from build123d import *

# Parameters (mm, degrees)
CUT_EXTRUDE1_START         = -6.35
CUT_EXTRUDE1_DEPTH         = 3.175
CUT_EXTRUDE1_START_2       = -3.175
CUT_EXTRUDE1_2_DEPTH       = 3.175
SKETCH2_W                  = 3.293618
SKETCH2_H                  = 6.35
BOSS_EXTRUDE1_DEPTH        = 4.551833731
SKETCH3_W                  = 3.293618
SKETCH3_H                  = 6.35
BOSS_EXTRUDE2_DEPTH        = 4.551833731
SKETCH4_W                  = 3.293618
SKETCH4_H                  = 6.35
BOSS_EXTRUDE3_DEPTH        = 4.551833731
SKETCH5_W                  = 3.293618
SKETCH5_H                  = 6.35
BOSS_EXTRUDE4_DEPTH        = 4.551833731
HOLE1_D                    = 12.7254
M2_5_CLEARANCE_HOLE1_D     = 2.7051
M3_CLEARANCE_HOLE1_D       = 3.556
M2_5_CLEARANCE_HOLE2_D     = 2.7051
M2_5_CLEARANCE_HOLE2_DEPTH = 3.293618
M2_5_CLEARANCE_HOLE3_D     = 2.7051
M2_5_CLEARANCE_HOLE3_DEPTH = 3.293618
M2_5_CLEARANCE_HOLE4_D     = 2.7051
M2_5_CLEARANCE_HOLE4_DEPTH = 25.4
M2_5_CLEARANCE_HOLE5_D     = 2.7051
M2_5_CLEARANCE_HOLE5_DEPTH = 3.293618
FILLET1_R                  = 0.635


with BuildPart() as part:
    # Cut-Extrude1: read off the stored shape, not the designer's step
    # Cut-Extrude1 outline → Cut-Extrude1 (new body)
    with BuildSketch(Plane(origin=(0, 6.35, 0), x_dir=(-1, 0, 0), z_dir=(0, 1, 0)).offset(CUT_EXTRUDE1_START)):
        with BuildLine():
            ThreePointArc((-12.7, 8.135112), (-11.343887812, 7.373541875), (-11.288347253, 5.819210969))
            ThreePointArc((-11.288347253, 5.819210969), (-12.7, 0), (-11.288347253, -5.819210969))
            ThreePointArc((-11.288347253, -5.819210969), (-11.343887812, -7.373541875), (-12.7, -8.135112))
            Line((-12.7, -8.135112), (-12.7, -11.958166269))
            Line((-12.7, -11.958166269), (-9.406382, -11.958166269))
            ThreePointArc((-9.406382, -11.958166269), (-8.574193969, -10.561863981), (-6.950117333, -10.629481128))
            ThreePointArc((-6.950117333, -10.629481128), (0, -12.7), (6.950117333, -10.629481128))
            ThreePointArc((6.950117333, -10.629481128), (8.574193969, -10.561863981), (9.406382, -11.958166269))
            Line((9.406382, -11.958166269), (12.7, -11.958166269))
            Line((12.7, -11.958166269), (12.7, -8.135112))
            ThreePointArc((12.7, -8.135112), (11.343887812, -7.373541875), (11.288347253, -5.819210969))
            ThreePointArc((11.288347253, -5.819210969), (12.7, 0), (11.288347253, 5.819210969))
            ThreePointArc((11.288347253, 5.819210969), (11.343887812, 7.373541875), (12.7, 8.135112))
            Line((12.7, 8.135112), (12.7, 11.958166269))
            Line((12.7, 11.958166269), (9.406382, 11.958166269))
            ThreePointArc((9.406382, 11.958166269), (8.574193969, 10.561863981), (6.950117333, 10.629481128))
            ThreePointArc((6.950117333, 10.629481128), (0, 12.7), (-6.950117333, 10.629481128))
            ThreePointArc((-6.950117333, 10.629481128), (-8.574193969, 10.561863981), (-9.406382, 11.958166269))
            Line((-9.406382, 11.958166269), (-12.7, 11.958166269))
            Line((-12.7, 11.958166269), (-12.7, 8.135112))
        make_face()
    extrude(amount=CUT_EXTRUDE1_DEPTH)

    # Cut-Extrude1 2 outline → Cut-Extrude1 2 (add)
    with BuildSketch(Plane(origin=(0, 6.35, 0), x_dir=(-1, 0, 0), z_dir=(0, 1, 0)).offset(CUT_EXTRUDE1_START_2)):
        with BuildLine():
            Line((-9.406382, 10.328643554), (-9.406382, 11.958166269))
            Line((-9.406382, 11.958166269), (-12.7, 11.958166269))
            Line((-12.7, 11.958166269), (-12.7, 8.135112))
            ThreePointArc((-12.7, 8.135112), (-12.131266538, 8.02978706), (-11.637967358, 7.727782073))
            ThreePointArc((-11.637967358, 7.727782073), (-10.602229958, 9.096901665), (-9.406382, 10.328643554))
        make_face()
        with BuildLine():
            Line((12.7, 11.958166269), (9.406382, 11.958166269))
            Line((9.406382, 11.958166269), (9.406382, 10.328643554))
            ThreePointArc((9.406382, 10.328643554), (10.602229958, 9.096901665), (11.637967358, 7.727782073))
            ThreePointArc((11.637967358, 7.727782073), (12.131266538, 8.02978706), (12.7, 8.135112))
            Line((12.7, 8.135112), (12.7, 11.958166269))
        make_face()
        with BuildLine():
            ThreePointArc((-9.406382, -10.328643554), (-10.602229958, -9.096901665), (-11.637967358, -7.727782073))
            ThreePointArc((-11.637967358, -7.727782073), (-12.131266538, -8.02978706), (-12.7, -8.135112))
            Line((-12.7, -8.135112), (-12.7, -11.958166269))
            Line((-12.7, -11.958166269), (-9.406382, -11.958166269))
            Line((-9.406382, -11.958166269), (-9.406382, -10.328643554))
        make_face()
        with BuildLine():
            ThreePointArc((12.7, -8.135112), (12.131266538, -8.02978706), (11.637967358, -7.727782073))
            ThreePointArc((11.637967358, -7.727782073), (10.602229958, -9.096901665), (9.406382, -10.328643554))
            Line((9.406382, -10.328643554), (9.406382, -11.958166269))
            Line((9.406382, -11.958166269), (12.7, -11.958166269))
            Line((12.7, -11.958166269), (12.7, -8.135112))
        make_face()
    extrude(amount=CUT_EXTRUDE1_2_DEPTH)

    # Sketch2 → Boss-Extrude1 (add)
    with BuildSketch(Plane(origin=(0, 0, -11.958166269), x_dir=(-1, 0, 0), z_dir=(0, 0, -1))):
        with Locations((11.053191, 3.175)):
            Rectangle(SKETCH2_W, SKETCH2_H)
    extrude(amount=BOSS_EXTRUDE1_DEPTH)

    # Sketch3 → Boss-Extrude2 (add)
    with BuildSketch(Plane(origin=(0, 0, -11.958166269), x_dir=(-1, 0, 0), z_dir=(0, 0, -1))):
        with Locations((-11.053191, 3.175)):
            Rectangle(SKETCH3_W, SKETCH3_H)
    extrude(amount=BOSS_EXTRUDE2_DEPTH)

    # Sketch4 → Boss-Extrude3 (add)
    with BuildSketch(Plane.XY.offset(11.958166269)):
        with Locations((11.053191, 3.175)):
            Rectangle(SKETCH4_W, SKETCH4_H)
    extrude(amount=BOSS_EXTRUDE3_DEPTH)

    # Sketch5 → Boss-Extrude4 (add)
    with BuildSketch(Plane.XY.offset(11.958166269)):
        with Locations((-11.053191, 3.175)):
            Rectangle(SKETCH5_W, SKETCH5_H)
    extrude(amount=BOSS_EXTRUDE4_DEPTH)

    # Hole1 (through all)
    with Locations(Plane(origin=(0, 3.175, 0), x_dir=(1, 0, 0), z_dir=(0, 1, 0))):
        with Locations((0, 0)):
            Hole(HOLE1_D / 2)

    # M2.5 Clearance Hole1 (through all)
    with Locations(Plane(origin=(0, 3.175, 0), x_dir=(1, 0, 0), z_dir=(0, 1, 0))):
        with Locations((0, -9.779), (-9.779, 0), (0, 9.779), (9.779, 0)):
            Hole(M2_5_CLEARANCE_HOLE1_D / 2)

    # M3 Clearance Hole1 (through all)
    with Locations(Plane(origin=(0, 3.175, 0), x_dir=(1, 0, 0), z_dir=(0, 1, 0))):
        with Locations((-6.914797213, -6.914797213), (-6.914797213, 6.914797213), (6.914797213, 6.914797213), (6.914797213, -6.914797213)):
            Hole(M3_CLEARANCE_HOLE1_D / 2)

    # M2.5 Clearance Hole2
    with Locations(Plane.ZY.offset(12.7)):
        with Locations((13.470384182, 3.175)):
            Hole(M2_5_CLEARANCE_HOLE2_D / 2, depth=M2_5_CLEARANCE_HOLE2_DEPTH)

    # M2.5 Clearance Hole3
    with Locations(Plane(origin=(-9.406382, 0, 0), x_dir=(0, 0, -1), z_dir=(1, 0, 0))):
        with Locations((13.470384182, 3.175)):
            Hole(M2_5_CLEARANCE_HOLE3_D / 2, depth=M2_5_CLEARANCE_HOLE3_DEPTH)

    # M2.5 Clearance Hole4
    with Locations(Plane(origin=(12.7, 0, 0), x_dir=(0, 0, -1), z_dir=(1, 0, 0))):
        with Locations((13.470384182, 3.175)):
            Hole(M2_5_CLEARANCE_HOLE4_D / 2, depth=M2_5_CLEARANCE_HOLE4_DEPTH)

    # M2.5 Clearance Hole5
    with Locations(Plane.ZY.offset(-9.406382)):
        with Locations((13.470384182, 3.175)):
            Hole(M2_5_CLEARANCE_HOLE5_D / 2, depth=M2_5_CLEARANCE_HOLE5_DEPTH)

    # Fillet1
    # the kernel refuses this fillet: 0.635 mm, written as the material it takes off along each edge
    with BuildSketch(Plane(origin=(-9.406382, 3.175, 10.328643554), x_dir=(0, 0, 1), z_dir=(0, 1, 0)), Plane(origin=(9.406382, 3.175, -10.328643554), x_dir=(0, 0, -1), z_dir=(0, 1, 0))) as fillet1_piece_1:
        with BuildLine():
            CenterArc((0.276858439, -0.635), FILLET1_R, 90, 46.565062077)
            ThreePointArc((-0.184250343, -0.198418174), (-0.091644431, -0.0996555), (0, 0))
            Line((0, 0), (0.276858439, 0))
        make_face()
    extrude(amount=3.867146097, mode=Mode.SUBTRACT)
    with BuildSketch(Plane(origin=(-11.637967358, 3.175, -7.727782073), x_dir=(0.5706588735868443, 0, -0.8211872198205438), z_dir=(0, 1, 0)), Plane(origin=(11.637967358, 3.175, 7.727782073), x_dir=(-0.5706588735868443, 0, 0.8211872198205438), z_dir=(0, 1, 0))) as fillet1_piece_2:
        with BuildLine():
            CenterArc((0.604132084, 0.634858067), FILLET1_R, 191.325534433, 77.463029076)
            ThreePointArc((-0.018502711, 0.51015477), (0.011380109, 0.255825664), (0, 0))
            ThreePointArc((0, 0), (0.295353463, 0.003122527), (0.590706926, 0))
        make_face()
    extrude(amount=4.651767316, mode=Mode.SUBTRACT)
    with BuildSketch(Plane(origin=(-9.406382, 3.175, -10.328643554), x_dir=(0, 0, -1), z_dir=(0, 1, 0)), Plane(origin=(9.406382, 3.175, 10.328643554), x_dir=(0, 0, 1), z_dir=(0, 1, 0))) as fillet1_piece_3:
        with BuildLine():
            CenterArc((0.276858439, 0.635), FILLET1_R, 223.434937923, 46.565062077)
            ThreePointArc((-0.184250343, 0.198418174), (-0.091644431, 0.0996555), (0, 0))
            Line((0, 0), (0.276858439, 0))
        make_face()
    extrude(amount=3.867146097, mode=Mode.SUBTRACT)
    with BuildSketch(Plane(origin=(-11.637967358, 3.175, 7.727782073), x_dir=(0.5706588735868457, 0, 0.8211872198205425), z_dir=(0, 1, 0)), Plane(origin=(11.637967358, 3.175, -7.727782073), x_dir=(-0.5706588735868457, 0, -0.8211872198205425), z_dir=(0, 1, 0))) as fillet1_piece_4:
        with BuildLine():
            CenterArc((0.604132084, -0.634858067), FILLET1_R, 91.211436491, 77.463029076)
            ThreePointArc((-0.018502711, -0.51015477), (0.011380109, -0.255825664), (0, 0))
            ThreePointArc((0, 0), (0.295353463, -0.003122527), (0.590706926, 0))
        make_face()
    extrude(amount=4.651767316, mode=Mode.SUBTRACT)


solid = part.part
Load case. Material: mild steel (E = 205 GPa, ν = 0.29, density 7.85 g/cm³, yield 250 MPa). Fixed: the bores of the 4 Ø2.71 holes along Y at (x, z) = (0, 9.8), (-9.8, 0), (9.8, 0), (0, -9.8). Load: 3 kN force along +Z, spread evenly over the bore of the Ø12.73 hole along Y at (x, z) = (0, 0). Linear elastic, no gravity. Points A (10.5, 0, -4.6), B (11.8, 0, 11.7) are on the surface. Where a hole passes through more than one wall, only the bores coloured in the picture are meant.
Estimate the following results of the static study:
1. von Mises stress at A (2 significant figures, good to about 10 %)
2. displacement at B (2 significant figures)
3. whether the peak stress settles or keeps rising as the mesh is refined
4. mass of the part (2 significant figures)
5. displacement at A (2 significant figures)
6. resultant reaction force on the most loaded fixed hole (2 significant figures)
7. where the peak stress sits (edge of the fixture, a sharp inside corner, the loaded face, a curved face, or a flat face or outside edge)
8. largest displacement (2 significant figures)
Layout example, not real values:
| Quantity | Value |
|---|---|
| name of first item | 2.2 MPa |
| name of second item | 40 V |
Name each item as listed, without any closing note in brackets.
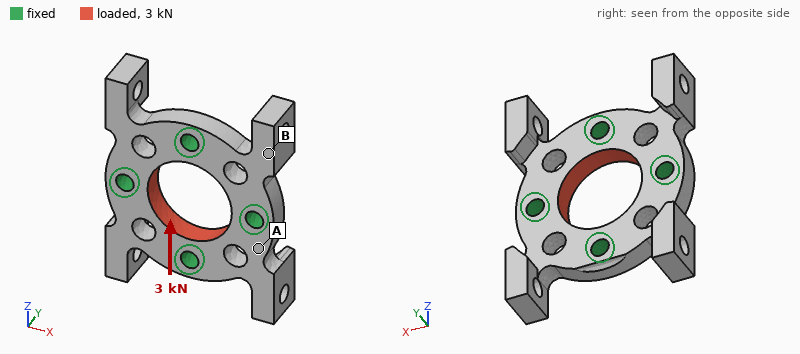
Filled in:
| Quantity | Value |
|---|---|
| von Mises stress at A | 19 MPa |
| displacement at B | 0.56 µm |
| whether the peak stress settles or keeps rising as the mesh is refined | keeps rising |
| mass of the part | 13 g |
| displacement at A | 0.61 µm |
| resultant reaction force on the most loaded fixed hole | 770 N |
| where the peak stress sits | edge of the fixture |
| largest displacement | 1.7 µm |
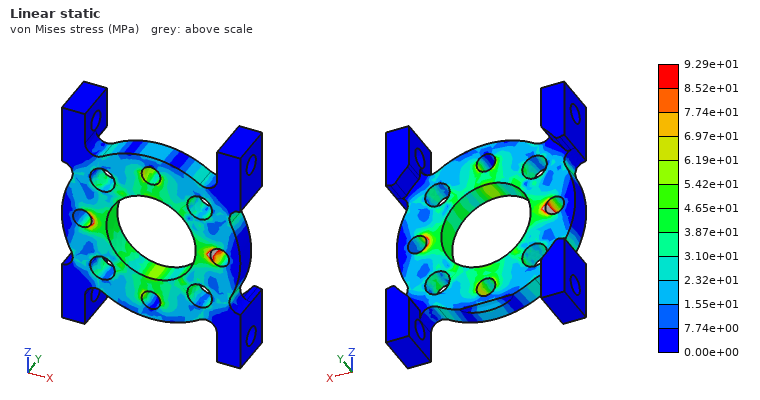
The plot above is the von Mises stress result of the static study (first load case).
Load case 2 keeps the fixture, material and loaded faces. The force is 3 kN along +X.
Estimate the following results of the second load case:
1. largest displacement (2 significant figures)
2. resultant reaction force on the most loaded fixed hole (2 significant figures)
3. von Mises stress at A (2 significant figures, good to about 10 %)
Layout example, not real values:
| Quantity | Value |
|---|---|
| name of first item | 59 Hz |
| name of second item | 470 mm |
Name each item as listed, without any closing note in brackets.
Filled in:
| Quantity | Value |
|---|---|
| largest displacement | 1.7 µm |
| resultant reaction force on the most loaded fixed hole | 760 N |
| von Mises stress at A | 17 MPa |
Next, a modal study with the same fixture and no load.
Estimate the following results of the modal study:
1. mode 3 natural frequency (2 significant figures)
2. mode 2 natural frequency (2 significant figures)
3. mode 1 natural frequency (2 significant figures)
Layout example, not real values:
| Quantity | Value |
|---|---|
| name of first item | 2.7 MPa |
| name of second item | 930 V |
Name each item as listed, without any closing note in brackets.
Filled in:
| Quantity | Value |
|---|---|
| mode 3 natural frequency | 12 kHz |
| mode 2 natural frequency | 12 kHz |
| mode 1 natural frequency | 12 kHz |
